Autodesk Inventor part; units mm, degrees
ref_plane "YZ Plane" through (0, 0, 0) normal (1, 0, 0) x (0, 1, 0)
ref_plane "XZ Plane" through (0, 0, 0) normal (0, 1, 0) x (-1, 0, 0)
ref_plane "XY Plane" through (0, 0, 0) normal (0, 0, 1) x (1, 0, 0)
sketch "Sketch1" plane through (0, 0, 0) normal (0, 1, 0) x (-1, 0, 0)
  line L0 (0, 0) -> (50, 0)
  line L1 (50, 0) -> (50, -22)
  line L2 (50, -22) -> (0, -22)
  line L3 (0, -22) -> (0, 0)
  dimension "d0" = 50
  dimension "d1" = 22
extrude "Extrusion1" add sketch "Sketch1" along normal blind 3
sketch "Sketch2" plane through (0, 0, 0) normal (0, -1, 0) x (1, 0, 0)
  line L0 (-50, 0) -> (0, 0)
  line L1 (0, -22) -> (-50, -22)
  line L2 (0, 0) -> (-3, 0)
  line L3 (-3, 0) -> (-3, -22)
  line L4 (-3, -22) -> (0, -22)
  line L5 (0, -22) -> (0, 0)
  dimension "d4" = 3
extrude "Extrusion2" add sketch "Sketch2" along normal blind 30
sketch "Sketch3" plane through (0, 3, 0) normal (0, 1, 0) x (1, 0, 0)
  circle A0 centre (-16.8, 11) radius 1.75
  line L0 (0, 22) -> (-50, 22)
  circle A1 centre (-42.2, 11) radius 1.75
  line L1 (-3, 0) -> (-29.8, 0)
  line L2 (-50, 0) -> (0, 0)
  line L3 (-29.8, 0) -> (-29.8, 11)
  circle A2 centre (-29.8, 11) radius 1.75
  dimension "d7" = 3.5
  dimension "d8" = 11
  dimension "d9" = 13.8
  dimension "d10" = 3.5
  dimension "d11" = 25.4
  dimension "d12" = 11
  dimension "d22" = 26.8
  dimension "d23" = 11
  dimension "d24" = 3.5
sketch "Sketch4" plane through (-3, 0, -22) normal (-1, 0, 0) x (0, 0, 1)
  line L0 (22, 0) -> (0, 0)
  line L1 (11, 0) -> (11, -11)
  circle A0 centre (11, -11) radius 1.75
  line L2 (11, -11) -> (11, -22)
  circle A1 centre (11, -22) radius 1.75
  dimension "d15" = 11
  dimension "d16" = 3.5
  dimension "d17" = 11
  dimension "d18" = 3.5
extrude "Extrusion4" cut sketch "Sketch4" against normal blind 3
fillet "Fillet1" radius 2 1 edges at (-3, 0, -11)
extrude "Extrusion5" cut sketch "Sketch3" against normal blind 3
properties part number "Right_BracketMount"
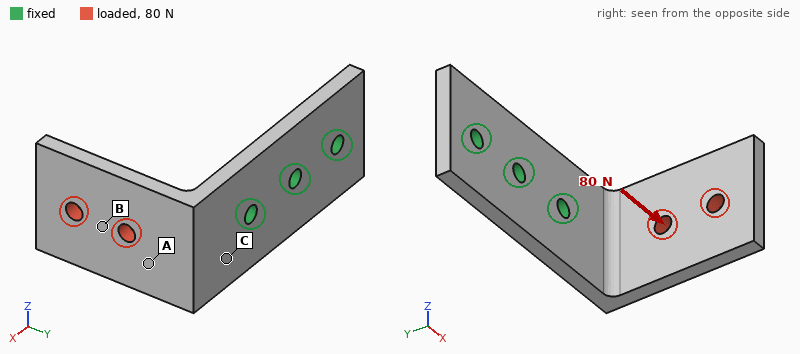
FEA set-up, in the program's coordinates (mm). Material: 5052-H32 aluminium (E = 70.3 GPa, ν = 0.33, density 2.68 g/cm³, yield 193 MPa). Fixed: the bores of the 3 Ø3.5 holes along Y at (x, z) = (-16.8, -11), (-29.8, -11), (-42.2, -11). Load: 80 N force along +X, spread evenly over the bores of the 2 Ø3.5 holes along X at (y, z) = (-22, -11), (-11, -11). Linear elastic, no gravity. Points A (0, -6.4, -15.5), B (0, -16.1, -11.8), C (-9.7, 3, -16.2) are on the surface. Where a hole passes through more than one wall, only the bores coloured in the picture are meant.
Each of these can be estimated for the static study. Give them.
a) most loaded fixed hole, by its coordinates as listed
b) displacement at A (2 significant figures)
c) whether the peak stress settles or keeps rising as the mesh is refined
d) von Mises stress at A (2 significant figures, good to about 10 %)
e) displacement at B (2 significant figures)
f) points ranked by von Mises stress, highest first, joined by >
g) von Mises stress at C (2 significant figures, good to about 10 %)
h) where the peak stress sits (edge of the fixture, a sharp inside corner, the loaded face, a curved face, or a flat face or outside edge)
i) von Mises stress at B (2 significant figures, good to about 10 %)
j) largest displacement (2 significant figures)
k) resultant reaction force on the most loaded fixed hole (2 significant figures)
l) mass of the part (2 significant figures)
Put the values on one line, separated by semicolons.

(-16.8, -11); 0.078 mm; keeps rising; 23 MPa; 0.15 mm; C > A > B; 38 MPa; edge of the fixture; 8.9 MPa; 0.27 mm; 74 N; 14 g
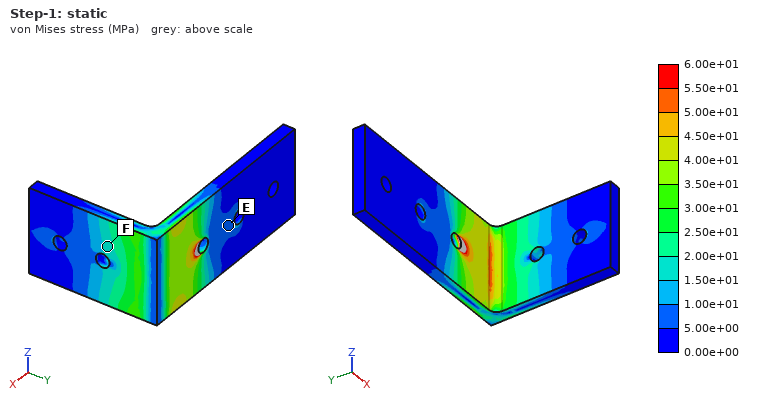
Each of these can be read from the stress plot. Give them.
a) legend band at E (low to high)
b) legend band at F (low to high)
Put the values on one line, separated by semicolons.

5.00e+00 to 1.00e+01 MPa; 1.50e+01 to 2.00e+01 MPa
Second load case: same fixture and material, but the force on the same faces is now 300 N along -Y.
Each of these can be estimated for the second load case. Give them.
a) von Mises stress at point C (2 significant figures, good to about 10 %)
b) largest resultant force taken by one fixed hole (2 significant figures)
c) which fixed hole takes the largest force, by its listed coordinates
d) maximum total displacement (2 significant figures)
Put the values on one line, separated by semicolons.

67 MPa; 420 N; (-16.8, -11); 0.33 mm
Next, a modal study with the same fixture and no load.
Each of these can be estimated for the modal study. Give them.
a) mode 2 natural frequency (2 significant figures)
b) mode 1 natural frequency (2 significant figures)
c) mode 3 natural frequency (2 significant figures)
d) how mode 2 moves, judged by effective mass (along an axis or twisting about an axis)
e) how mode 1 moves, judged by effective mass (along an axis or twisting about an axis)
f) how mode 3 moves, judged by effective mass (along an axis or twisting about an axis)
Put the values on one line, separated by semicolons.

2200 Hz; 1500 Hz; 5100 Hz; along Z; along X; along Y
